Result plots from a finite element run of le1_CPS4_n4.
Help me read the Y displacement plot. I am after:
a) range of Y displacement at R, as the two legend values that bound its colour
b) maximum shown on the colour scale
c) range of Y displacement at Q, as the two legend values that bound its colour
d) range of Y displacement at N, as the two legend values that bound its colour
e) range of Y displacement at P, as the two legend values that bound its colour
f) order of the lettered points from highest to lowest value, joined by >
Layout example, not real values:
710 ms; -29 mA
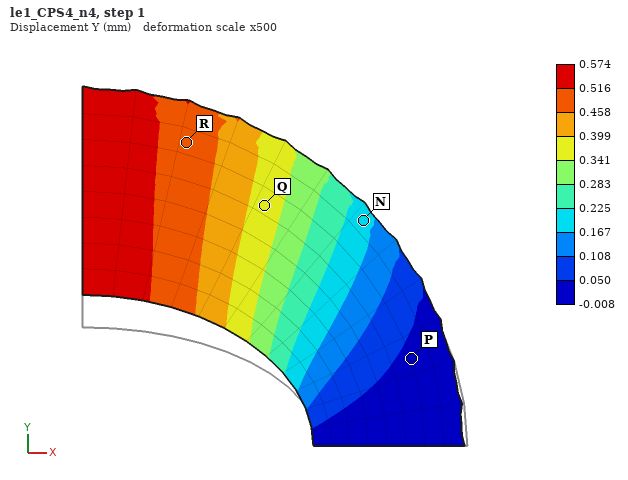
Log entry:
0.458 to 0.516 mm; 0.574 mm; 0.341 to 0.399 mm; 0.167 to 0.225 mm; -0.008 to 0.050 mm; R > Q > N > P
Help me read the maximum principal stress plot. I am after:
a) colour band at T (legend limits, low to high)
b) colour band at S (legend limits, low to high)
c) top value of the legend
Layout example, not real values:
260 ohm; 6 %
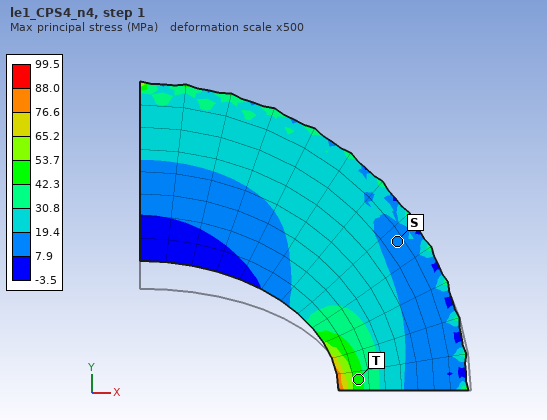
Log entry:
42.3 to 53.7 MPa; 7.9 to 19.4 MPa; 99.5 MPa
